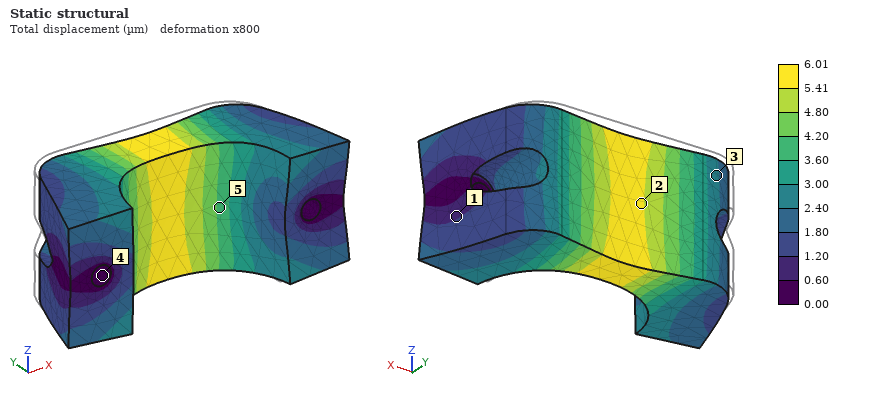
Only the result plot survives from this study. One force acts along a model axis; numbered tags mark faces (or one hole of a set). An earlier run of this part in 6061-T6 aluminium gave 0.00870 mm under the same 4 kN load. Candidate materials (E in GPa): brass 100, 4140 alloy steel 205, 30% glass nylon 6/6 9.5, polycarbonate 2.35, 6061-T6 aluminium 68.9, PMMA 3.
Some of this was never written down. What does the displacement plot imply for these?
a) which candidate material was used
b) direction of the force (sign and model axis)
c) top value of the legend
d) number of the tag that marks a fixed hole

brass
-Y
6.01 µm
4
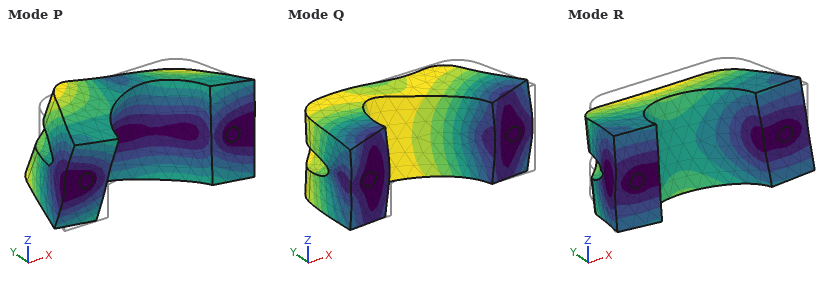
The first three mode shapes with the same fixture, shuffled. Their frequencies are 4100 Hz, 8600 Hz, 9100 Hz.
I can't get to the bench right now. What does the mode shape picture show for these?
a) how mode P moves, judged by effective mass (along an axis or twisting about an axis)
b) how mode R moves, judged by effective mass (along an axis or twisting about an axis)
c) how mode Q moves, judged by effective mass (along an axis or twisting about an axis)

twisting about Y
along Z
along X
